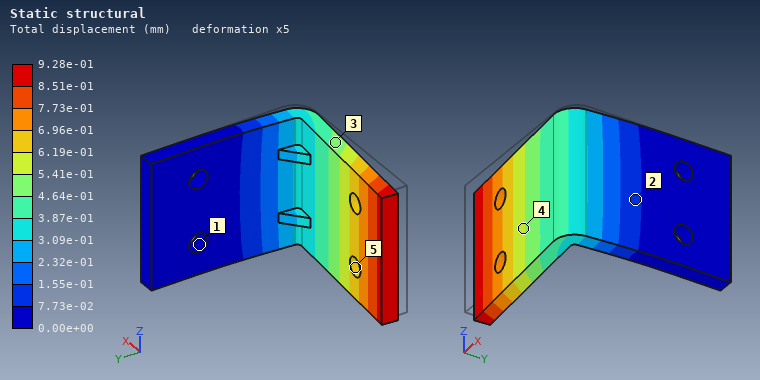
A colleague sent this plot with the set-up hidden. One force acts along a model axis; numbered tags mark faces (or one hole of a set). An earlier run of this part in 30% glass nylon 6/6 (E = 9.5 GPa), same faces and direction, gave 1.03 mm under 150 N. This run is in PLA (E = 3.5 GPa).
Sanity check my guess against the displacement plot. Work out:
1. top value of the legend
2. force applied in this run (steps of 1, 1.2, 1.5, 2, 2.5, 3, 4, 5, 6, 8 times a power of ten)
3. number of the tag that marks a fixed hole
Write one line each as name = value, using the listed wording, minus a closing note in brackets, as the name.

top value of the legend = 9.28e-01 mm
force applied in this run = 50 N
number of the tag that marks a fixed hole = 1
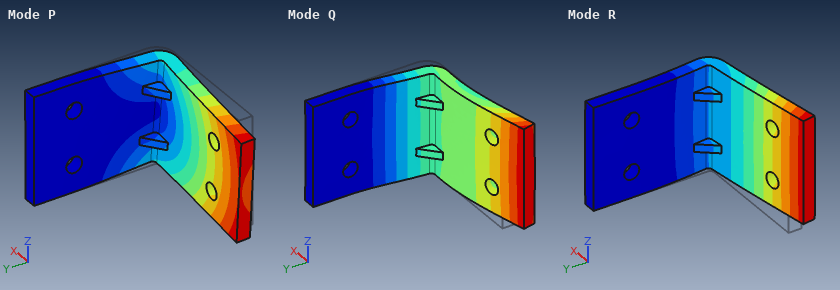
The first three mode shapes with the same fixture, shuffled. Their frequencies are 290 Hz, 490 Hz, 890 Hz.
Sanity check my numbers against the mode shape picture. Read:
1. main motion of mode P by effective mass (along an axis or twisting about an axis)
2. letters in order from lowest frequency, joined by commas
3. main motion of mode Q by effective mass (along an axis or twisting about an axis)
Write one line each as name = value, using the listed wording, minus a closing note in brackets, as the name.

main motion of mode P by effective mass = along Z
letters in order from lowest frequency, joined by commas = R, P, Q
main motion of mode Q by effective mass = along X
